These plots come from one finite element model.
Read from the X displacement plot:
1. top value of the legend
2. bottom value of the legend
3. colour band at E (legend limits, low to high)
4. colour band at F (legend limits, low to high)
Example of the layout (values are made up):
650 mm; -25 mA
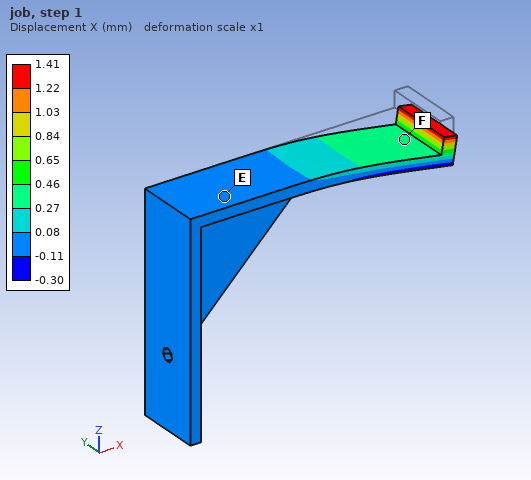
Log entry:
1.41 mm; -0.30 mm; -0.11 to 0.08 mm; 0.27 to 0.46 mm
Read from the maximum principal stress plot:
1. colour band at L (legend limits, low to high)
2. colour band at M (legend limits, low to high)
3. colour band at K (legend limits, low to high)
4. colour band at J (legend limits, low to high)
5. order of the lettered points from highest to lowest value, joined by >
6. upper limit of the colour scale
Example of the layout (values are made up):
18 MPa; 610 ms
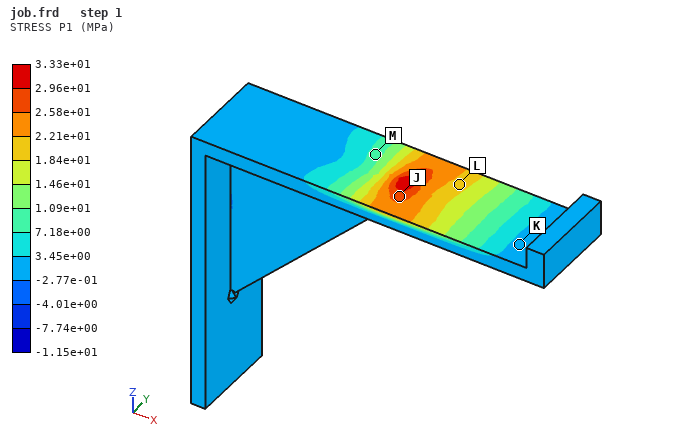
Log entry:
1.84e+01 to 2.21e+01 MPa; 7.18e+00 to 1.09e+01 MPa; -2.77e-01 to 3.45e+00 MPa; 2.58e+01 to 2.96e+01 MPa; J > L > M > K; 3.33e+01 MPa
